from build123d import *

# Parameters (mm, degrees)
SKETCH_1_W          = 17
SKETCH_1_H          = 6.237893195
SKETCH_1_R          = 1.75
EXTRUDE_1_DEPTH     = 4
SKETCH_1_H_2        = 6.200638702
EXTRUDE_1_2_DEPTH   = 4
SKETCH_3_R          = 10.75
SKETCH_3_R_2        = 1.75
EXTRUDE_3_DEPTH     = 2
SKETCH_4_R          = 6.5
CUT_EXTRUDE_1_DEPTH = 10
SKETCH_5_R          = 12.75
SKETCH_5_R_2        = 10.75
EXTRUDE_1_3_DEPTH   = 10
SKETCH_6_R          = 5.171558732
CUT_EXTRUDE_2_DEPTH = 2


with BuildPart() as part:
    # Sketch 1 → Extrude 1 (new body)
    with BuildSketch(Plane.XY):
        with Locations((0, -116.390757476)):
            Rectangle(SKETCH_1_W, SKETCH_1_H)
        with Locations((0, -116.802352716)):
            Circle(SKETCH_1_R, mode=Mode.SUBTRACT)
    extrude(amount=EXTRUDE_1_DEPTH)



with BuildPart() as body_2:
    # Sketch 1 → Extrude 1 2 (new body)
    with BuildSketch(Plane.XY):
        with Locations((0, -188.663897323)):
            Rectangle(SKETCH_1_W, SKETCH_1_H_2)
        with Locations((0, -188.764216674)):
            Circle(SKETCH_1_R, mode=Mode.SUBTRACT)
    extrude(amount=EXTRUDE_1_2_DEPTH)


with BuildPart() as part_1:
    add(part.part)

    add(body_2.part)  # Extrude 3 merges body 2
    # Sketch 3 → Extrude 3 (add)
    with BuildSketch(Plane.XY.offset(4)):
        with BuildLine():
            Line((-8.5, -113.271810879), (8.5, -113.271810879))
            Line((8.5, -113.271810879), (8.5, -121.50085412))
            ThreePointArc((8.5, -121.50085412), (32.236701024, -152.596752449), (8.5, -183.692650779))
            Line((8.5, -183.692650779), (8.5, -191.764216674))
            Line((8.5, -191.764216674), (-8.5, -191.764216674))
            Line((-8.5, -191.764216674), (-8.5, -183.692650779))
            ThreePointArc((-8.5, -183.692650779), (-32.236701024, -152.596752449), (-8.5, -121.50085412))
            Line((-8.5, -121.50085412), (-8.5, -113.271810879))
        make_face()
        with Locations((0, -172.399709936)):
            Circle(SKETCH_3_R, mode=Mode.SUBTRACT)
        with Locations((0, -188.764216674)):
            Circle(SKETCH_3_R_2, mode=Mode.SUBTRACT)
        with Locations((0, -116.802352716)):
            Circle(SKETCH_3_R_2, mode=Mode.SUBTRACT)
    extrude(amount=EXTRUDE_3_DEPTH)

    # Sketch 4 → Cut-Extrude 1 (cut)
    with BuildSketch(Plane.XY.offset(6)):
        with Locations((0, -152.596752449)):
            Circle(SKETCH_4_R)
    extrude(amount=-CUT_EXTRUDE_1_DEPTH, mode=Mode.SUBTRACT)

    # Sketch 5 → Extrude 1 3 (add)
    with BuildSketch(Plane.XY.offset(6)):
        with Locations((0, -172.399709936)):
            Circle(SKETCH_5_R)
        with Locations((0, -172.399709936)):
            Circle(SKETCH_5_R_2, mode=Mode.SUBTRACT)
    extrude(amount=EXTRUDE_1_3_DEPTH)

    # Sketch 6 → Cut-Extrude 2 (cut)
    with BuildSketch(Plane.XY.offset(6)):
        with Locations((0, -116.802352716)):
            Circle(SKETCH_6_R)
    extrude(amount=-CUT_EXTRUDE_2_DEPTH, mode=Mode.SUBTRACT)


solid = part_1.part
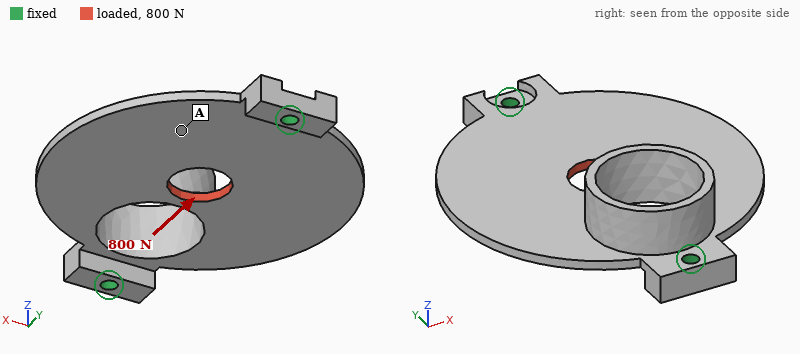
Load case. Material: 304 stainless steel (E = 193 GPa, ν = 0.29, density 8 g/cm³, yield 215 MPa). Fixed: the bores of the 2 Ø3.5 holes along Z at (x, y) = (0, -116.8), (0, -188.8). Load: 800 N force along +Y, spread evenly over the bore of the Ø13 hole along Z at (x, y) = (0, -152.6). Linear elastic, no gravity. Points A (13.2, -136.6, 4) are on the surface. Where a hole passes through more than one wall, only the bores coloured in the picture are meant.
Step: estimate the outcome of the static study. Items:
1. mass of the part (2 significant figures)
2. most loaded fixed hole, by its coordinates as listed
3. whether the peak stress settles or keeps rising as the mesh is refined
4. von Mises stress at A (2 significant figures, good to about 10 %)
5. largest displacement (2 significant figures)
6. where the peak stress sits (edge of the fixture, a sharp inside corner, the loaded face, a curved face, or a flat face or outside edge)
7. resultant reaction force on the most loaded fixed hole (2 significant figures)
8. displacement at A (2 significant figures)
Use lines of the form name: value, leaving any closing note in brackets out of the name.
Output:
mass of the part: 65 g
most loaded fixed hole, by its coordinates as listed: (0, -116.8)
whether the peak stress settles or keeps rising as the mesh is refined: keeps rising
von Mises stress at A: 7.5 MPa
largest displacement: 8.2 µm
where the peak stress sits: edge of the fixture
resultant reaction force on the most loaded fixed hole: 440 N
displacement at A: 6.6 µm
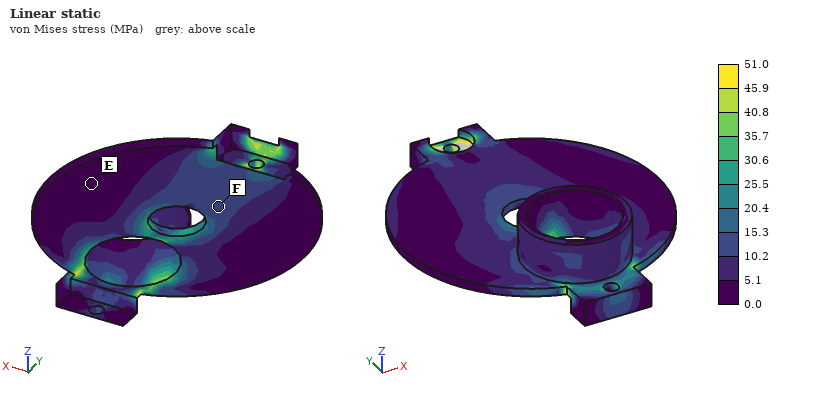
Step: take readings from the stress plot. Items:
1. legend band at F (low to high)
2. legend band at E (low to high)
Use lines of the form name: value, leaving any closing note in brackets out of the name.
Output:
legend band at F: 10.2 to 15.3 MPa
legend band at E: 0.0 to 5.1 MPa
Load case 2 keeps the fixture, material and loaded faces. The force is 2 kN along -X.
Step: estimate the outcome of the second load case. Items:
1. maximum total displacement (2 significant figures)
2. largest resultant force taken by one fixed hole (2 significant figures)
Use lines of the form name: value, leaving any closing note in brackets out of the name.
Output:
maximum total displacement: 17 µm
largest resultant force taken by one fixed hole: 1.0 kN
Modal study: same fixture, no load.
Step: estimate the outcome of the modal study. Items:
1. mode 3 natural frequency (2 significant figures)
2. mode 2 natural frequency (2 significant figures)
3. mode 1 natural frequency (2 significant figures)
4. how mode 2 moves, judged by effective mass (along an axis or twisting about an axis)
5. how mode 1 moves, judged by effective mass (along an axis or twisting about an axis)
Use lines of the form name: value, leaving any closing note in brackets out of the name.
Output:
mode 3 natural frequency: 3700 Hz
mode 2 natural frequency: 1600 Hz
mode 1 natural frequency: 1400 Hz
how mode 2 moves, judged by effective mass: twisting about Y
how mode 1 moves, judged by effective mass: along Z
